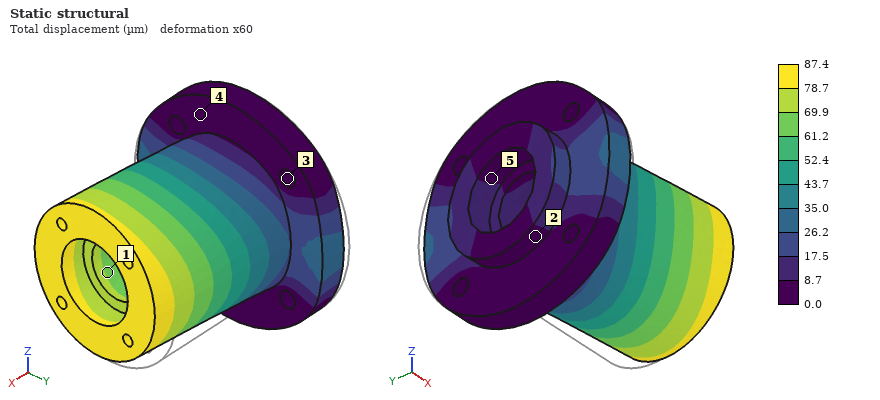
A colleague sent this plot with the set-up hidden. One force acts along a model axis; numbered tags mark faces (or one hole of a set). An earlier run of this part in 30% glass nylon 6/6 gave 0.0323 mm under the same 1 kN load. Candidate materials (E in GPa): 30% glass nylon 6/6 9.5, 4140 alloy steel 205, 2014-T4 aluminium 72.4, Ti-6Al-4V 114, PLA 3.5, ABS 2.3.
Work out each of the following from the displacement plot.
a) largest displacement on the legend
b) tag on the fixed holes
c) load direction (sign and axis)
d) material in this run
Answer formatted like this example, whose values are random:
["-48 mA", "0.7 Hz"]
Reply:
["87.4 µm", "3", "-Y", "PLA"]
